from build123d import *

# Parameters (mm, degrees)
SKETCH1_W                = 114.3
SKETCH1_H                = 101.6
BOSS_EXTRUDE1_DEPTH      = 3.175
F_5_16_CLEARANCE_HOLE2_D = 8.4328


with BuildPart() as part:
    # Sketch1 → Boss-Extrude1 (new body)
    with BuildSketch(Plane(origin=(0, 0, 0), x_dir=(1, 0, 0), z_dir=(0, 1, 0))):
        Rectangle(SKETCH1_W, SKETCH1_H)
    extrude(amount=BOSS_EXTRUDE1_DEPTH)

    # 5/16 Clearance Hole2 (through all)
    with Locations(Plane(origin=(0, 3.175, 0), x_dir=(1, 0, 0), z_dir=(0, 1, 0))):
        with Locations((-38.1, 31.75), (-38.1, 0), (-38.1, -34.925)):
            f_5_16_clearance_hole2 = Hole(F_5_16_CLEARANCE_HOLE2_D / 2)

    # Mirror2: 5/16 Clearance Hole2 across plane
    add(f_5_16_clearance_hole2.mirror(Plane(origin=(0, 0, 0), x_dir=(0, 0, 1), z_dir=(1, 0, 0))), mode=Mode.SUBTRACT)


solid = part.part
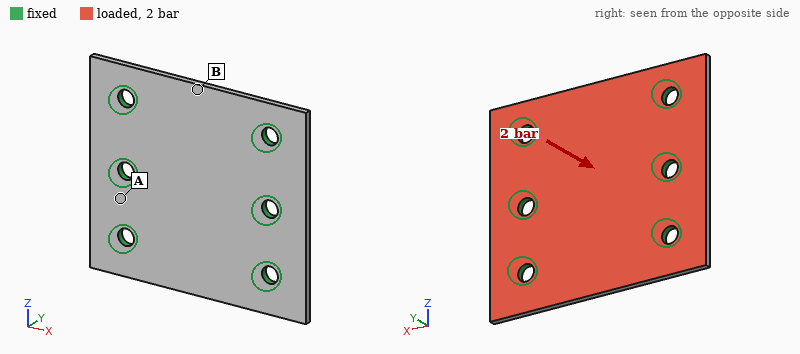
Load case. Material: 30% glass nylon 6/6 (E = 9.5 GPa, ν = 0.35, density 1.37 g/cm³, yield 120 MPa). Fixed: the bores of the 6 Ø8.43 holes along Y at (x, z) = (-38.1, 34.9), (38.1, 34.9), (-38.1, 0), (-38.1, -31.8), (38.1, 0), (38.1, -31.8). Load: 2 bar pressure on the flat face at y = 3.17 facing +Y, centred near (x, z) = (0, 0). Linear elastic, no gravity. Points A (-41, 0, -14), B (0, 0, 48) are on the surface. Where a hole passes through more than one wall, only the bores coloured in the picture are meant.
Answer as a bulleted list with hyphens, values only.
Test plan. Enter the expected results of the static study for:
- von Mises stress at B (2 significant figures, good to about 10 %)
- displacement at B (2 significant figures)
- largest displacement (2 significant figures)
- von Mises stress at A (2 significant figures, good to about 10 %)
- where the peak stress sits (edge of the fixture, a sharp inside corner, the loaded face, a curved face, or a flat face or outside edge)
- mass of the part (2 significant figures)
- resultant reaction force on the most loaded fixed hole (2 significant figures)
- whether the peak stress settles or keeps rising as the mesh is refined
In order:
- 26 MPa
- 0.61 mm
- 0.72 mm
- 12 MPa
- edge of the fixture
- 49 g
- 400 N
- keeps rising
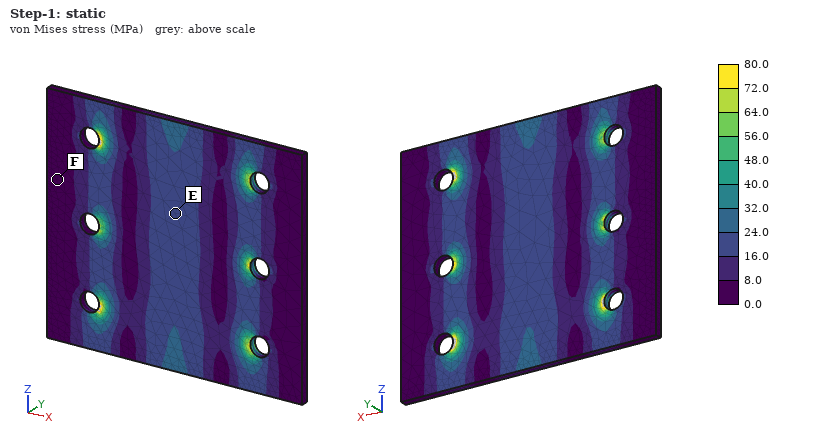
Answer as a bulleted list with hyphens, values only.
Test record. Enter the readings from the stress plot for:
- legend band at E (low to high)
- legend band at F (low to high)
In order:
- 16.0 to 24.0 MPa
- 0.0 to 8.0 MPa
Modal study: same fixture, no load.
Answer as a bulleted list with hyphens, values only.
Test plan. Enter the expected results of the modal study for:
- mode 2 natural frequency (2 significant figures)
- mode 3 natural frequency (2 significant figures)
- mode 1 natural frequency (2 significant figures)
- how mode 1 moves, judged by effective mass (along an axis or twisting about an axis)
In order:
- 1700 Hz
- 2300 Hz
- 1600 Hz
- along Y
